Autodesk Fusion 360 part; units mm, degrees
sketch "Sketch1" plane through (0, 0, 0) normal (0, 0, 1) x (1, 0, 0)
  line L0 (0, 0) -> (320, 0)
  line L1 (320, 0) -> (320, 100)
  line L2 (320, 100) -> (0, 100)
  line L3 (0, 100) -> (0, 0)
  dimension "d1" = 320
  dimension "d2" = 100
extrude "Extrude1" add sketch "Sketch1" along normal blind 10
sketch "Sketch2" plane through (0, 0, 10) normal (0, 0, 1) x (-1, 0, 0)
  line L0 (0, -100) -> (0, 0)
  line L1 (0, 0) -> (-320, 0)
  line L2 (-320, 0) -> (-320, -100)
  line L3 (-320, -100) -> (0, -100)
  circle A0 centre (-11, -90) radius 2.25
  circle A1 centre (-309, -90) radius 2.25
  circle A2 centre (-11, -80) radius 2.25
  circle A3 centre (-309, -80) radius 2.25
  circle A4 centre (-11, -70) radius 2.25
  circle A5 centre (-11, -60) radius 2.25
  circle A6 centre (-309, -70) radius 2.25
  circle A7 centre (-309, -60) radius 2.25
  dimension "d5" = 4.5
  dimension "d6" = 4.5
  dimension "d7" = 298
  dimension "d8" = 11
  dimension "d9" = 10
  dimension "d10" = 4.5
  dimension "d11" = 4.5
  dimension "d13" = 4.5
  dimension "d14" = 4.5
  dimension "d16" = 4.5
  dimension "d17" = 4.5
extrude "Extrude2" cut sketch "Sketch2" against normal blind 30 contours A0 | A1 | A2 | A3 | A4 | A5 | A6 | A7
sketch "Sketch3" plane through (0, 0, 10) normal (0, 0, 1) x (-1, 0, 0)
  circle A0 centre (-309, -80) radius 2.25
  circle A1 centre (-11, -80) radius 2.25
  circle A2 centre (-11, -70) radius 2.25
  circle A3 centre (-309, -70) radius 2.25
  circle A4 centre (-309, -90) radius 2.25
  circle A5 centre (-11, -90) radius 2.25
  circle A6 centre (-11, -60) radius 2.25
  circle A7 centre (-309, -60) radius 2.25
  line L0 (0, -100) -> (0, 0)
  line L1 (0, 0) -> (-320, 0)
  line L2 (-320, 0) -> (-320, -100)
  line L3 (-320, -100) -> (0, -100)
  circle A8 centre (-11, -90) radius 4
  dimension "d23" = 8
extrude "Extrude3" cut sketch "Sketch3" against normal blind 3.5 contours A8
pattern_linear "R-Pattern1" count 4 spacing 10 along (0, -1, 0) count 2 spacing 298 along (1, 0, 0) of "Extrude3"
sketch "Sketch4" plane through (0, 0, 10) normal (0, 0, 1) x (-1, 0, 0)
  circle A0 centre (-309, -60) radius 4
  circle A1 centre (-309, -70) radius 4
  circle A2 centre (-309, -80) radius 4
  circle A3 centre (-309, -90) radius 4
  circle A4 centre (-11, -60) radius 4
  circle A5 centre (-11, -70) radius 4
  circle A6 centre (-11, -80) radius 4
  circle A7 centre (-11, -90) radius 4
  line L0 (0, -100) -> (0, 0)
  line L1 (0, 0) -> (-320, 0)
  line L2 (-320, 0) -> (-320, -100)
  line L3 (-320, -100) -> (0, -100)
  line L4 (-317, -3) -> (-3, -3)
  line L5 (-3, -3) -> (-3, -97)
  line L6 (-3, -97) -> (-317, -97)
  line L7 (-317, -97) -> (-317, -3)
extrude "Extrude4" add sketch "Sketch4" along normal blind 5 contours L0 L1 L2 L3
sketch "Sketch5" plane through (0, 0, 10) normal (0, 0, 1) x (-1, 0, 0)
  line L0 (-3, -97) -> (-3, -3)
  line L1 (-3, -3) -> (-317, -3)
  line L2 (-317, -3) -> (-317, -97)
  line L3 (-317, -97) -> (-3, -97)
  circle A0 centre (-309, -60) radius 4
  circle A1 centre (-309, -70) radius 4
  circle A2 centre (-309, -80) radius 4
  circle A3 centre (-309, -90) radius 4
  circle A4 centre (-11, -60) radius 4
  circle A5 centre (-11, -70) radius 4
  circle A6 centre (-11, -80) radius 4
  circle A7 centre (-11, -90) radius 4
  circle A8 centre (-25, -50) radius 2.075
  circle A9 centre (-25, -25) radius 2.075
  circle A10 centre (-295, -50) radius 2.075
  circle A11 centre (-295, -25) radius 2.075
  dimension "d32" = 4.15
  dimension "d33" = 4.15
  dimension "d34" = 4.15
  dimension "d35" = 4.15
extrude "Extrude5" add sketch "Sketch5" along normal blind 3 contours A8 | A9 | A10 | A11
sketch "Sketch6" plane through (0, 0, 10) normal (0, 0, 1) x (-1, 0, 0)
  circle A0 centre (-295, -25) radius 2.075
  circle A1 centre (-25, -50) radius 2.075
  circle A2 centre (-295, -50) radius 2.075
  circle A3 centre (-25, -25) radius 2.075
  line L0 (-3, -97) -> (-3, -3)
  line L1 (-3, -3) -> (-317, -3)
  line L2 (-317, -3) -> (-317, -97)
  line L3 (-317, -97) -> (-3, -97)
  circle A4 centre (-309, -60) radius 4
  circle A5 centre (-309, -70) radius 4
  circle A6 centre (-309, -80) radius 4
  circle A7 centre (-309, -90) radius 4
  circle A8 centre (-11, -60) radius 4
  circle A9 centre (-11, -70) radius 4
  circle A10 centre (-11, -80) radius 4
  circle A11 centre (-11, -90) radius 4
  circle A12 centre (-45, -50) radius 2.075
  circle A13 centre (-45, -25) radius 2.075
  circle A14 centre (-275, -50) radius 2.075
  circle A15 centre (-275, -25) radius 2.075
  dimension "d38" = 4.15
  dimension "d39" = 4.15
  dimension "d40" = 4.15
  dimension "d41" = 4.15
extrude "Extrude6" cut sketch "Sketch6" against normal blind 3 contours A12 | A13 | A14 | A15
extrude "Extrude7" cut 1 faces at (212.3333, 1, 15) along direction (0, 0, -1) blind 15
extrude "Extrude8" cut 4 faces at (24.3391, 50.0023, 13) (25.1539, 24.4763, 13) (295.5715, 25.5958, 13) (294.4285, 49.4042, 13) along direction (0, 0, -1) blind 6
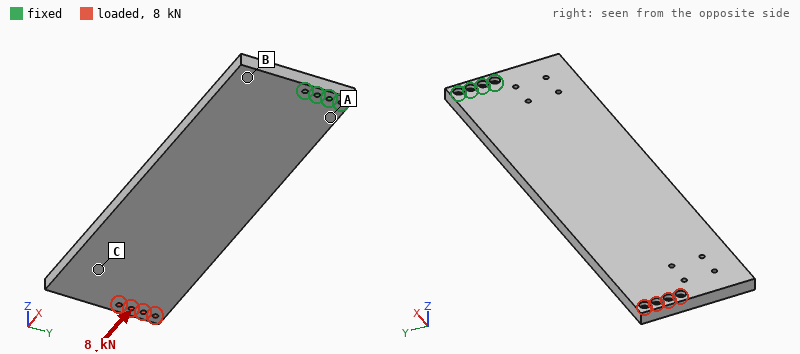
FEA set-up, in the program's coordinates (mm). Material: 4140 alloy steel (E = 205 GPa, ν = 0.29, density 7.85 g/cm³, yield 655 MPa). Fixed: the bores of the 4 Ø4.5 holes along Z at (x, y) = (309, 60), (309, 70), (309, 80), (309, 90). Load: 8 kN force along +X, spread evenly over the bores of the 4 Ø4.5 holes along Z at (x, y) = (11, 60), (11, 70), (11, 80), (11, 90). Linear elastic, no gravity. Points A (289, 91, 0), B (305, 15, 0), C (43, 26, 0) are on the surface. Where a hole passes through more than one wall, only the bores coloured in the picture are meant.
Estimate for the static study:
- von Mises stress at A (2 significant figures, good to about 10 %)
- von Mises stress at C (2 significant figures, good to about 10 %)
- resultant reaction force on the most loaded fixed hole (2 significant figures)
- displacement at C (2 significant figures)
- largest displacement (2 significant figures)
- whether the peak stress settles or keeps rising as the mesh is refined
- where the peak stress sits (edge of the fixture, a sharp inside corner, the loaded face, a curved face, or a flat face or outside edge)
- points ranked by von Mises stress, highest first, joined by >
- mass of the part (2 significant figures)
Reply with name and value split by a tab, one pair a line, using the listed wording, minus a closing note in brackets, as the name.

von Mises stress at A	32 MPa
von Mises stress at C	8.0 MPa
resultant reaction force on the most loaded fixed hole	2.4 kN
displacement at C	0.33 mm
largest displacement	0.44 mm
whether the peak stress settles or keeps rising as the mesh is refined	keeps rising
where the peak stress sits	edge of the fixture
points ranked by von Mises stress, highest first, joined by >	A > C > B
mass of the part	2.3 kg
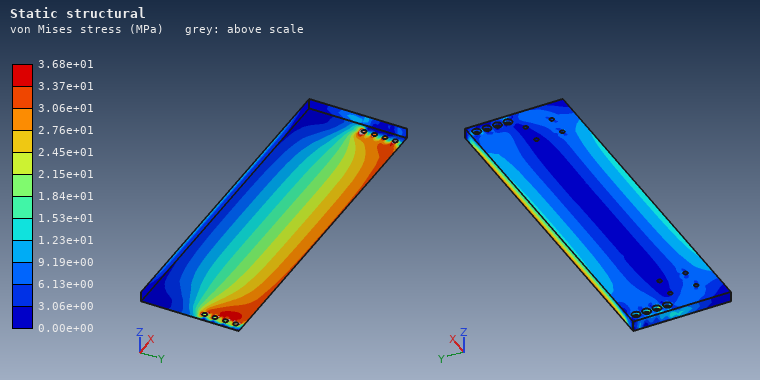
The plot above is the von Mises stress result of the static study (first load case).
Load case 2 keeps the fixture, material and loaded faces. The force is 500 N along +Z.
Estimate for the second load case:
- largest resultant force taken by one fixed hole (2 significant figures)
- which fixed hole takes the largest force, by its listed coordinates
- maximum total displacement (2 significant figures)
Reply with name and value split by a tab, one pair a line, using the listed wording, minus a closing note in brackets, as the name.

largest resultant force taken by one fixed hole	1.2 kN
which fixed hole takes the largest force, by its listed coordinates	(309, 70)
maximum total displacement	3.6 mm
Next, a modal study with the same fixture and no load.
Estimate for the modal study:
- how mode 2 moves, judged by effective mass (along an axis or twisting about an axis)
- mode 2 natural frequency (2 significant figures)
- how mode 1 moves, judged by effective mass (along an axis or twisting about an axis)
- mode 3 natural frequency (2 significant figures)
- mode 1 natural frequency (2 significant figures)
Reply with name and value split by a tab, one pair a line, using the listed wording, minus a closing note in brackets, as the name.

how mode 2 moves, judged by effective mass	along Y
mode 2 natural frequency	410 Hz
how mode 1 moves, judged by effective mass	along Z
mode 3 natural frequency	470 Hz
mode 1 natural frequency	77 Hz
